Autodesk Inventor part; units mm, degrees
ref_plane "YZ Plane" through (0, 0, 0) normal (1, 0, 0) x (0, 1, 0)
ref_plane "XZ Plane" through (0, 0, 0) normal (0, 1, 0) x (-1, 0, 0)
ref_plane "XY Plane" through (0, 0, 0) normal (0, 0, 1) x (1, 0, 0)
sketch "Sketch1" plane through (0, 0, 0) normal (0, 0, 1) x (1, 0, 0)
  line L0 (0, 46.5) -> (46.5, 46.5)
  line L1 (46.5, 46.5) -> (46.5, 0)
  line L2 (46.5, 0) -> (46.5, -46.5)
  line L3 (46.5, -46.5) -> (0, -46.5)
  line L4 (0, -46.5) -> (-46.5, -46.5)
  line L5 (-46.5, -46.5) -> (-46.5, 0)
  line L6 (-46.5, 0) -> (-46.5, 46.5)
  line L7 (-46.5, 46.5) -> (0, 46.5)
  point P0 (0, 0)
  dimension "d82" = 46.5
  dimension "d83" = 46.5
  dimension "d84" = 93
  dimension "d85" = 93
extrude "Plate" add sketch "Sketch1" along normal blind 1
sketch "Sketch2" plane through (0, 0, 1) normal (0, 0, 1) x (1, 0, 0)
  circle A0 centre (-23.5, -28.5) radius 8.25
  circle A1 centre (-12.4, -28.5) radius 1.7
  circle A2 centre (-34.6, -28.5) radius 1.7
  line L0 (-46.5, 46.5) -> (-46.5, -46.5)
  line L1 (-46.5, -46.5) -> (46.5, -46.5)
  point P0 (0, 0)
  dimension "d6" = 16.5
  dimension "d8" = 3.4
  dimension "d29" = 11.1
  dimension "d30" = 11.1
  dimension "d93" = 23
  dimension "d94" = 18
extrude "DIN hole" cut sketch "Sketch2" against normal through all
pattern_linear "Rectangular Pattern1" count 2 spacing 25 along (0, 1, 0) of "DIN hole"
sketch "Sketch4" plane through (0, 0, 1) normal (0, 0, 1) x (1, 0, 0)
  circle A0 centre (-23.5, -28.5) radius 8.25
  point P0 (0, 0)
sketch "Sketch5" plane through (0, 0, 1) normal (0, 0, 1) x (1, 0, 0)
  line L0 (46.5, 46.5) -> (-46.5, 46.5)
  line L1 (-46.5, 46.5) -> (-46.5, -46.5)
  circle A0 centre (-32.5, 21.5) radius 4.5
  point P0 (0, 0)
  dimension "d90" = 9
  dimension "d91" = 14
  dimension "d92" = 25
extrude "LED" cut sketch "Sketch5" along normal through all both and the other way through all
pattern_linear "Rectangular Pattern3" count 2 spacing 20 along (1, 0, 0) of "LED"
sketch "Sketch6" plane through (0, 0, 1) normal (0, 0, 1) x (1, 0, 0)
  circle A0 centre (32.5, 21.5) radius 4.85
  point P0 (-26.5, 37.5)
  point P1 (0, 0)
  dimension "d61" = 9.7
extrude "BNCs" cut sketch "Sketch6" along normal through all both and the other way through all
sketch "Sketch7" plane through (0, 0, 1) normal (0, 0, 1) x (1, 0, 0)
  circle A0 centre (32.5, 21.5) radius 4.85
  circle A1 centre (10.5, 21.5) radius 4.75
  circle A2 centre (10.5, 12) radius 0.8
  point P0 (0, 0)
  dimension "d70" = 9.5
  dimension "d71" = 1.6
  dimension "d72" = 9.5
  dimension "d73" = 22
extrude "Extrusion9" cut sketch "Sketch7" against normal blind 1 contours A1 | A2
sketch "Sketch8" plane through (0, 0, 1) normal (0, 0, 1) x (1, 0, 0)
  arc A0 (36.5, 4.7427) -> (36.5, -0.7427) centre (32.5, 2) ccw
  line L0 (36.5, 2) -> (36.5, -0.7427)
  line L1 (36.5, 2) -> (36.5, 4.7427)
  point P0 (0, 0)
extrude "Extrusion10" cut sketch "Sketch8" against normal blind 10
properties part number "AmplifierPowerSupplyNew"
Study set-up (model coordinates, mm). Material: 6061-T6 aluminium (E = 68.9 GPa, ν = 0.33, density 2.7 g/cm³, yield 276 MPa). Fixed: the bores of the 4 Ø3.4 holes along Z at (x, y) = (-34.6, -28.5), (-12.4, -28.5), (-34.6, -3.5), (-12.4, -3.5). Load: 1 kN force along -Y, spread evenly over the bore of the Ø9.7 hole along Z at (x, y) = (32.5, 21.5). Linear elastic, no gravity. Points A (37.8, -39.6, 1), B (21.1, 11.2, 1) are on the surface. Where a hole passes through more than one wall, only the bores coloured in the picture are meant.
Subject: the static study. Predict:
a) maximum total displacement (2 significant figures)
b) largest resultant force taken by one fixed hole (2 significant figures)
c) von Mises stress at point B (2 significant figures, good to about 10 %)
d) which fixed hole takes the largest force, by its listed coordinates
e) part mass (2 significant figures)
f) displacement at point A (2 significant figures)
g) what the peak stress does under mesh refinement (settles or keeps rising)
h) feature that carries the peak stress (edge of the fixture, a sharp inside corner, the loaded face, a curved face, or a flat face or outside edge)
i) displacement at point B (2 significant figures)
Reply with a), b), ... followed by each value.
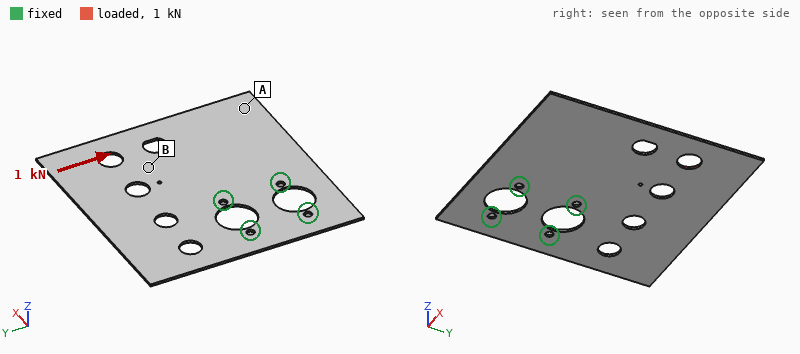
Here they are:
a) 0.14 mm
b) 1.2 kN
c) 31 MPa
d) (-12.4, -3.5)
e) 21 g
f) 0.087 mm
g) keeps rising
h) edge of the fixture
i) 0.072 mm
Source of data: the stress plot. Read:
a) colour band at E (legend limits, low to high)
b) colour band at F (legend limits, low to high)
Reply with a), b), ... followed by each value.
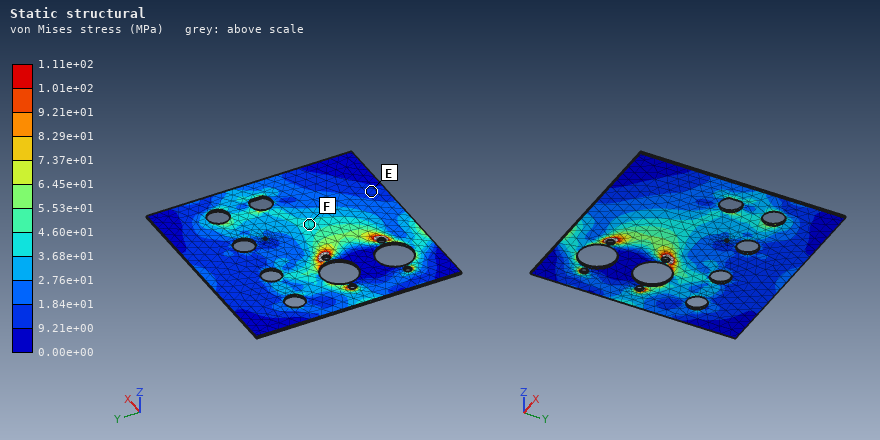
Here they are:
a) 9.21e+00 to 1.84e+01 MPa
b) 3.68e+01 to 4.60e+01 MPa
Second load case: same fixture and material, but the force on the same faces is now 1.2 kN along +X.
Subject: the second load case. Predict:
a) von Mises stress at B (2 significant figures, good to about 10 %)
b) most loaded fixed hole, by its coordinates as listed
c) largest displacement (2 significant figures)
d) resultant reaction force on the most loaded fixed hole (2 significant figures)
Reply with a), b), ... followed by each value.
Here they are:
a) 46 MPa
b) (-12.4, -3.5)
c) 0.11 mm
d) 1.2 kN
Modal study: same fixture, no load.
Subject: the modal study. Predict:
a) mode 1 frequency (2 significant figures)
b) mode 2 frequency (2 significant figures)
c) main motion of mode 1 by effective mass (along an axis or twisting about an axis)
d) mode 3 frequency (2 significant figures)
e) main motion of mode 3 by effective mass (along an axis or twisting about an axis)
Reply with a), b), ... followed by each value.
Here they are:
a) 200 Hz
b) 270 Hz
c) along Z
d) 440 Hz
e) along Z
